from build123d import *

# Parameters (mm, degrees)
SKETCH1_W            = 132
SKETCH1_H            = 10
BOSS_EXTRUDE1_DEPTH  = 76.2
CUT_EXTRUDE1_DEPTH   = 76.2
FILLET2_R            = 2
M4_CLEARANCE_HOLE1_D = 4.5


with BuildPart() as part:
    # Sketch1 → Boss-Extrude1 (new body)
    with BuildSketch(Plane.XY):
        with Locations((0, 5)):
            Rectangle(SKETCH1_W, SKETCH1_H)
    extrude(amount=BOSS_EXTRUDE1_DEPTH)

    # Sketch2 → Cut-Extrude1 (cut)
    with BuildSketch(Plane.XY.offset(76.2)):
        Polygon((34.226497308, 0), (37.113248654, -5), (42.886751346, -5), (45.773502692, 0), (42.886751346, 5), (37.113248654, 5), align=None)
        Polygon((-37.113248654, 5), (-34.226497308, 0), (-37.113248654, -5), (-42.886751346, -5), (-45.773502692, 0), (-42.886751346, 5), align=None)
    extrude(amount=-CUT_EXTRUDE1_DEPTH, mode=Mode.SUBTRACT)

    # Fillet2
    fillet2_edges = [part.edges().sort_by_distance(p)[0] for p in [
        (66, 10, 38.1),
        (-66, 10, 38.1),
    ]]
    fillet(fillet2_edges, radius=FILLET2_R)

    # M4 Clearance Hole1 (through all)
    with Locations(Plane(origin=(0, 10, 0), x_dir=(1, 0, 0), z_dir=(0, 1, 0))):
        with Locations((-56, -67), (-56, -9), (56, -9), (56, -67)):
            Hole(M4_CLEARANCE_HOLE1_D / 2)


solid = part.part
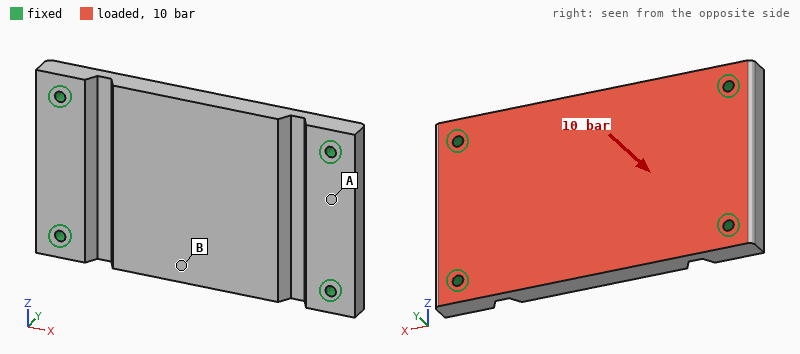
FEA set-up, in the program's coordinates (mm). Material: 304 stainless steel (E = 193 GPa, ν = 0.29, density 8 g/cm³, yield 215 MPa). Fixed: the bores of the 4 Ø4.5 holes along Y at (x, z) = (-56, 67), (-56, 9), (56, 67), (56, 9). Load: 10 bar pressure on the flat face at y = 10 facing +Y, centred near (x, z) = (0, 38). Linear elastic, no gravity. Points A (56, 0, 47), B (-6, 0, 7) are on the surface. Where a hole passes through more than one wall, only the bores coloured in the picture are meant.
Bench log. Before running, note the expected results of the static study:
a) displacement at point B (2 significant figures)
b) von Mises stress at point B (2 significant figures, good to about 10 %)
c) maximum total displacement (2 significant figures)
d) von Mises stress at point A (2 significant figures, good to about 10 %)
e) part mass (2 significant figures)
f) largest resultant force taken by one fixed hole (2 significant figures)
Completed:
43 µm
45 MPa
45 µm
17 MPa
750 g
2.5 kN
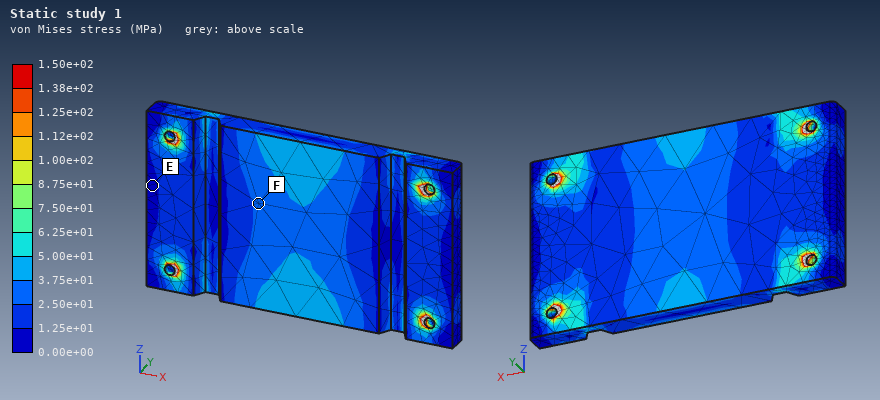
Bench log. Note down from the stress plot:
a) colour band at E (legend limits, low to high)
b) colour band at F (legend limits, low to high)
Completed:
0.00e+00 to 1.25e+01 MPa
2.50e+01 to 3.75e+01 MPa
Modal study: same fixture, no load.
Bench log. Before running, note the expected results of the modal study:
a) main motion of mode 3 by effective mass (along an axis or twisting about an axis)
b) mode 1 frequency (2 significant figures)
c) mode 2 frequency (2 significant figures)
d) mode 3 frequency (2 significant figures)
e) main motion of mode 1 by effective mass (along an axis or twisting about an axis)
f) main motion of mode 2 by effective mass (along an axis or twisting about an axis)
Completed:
twisting about Z
3100 Hz
4400 Hz
7700 Hz
along Y
twisting about X
